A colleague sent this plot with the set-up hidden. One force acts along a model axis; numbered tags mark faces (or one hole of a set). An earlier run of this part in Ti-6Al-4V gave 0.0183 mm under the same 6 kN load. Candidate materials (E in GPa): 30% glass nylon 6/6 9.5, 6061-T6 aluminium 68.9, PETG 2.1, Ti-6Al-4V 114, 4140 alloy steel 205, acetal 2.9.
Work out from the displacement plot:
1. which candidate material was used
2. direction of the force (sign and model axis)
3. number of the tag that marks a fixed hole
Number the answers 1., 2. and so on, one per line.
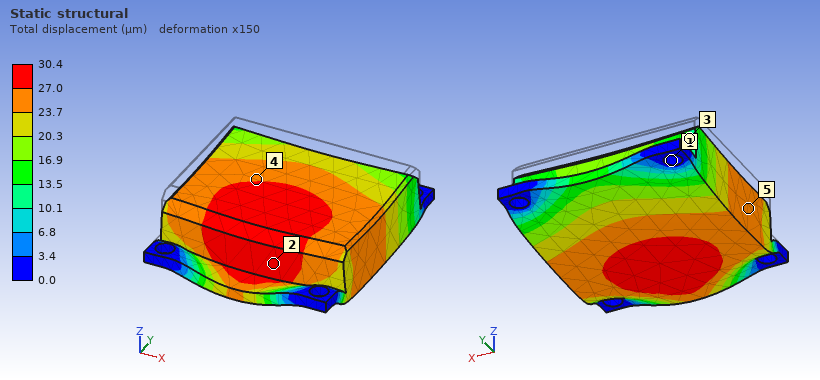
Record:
1. 6061-T6 aluminium
2. -Z
3. 1
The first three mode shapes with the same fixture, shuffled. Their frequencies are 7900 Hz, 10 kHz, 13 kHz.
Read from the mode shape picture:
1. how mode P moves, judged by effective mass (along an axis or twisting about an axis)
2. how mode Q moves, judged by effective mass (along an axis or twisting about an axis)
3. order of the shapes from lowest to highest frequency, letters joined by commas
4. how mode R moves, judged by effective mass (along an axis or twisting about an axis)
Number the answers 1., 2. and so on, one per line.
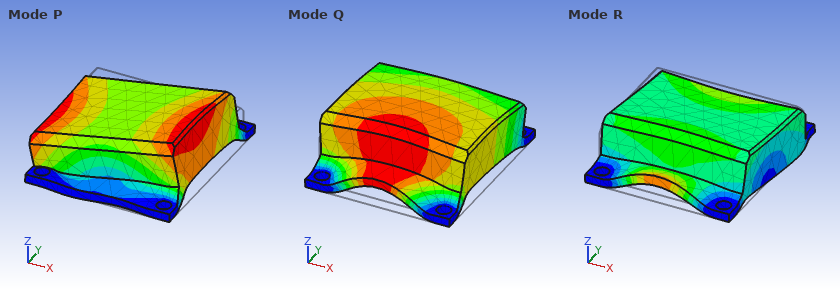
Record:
1. along X
2. along Z
3. Q, P, R
4. along Y
